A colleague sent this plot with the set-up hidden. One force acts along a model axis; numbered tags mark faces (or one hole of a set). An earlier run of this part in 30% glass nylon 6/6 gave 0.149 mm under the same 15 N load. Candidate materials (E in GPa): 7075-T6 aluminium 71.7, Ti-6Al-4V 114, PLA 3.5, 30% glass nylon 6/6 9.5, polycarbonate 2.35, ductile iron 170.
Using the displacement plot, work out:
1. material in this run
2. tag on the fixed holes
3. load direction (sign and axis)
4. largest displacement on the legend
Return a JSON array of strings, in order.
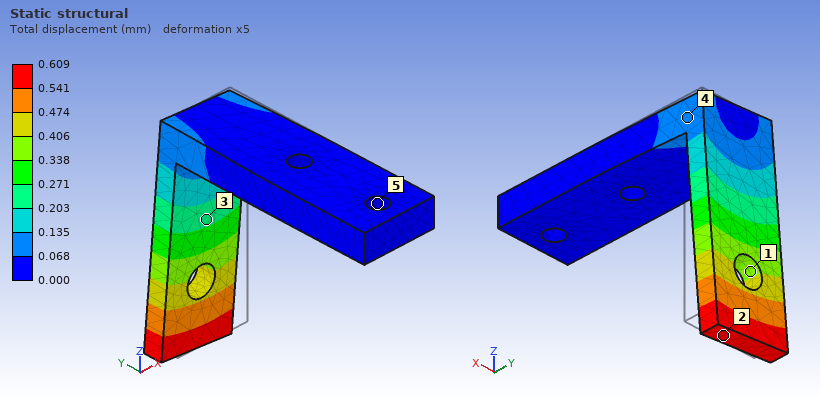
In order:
["polycarbonate", "5", "-X", "0.609 mm"]
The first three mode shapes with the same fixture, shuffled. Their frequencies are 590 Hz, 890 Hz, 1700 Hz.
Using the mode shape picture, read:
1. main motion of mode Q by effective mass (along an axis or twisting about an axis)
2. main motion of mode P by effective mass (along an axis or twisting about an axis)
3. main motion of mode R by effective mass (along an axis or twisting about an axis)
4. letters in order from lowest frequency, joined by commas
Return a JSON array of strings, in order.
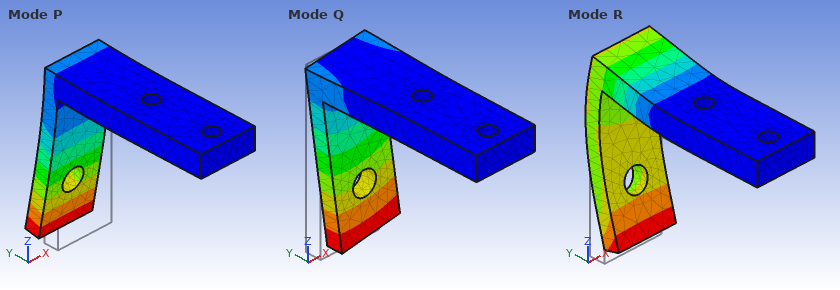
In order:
["along X", "along Y", "along Z", "P, Q, R"]
